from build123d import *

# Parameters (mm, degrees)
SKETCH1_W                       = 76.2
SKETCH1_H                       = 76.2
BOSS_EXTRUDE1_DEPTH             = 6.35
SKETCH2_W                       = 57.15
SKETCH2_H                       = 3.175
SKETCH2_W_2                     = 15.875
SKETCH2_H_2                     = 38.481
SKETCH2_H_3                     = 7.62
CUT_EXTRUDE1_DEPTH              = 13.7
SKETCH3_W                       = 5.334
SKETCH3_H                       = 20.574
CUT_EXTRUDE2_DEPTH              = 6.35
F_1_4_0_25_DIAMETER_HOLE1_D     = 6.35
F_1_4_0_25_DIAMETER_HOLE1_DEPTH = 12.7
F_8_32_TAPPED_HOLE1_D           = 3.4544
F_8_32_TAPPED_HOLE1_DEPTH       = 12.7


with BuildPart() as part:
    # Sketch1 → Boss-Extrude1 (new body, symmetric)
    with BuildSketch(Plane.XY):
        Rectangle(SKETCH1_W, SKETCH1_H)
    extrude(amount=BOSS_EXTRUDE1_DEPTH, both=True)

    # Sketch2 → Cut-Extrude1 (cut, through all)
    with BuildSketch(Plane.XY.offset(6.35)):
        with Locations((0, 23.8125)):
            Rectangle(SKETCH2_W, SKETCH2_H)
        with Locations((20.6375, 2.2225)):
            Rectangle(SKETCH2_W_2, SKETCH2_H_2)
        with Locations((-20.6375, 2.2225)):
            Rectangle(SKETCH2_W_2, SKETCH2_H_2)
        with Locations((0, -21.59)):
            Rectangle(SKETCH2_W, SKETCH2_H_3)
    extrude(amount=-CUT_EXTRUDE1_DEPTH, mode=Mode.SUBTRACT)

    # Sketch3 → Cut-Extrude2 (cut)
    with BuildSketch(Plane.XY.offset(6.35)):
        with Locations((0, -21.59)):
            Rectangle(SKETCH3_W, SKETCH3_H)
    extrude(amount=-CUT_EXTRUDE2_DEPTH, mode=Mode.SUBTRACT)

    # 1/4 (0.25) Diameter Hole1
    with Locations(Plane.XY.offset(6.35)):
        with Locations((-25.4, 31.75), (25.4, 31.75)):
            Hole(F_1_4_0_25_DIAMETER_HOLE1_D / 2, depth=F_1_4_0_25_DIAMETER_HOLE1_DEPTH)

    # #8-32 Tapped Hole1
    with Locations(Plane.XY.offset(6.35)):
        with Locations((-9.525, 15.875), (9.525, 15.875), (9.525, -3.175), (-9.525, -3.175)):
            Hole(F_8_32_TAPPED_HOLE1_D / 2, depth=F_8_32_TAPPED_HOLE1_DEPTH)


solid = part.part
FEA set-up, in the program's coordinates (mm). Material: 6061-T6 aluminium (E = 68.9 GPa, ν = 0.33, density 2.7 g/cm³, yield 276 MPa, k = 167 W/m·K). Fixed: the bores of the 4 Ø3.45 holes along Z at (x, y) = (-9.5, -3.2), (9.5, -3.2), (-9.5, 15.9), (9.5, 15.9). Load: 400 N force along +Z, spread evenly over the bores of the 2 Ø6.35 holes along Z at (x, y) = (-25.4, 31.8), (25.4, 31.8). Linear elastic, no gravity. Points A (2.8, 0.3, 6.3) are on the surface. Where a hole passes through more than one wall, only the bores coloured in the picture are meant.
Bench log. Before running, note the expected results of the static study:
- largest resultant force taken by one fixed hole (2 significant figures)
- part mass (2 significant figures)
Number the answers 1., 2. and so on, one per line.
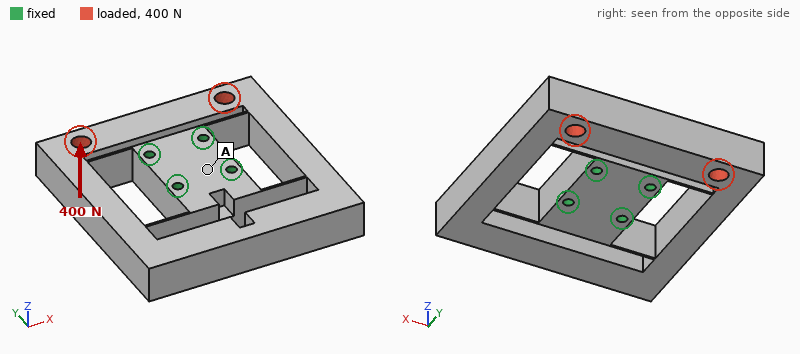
1. 270 N
2. 130 g
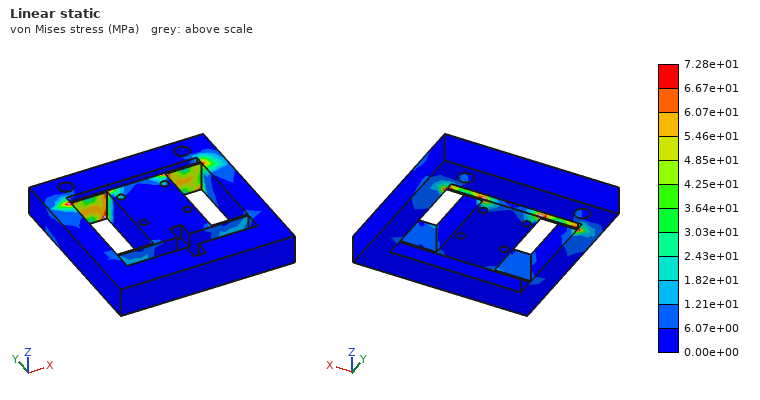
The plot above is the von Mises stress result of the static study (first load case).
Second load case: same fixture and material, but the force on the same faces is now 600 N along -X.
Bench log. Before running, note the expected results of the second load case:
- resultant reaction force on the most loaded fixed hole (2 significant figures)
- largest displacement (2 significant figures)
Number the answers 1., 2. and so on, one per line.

1. 400 N
2. 36 µm
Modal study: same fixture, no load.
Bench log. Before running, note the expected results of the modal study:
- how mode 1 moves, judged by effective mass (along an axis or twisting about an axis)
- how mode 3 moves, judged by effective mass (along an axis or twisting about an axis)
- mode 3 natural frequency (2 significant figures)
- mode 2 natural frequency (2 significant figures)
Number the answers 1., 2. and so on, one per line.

1. along Y
2. twisting about Z
3. 1700 Hz
4. 1600 Hz
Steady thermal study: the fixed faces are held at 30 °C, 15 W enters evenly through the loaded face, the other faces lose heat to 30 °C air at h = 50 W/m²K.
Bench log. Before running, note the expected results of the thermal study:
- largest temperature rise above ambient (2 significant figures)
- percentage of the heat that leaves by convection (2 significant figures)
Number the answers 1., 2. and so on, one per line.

1. 21 K
2. 67 %
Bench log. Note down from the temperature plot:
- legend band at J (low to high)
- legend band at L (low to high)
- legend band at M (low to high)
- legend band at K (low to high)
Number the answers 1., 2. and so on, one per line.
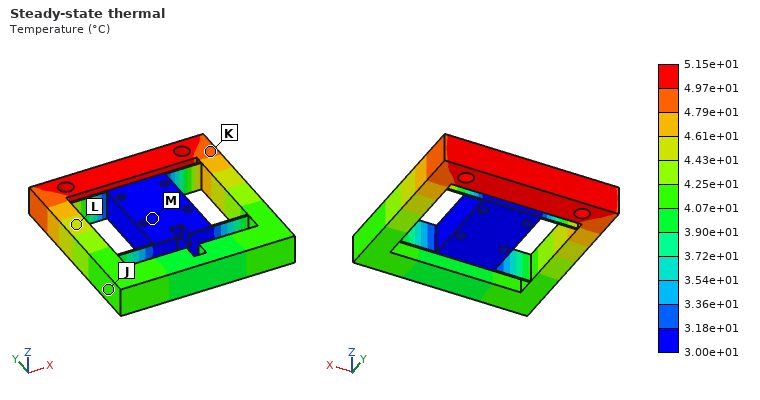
1. 4.07e+01 to 4.25e+01 °C
2. 4.43e+01 to 4.61e+01 °C
3. 3.00e+01 to 3.18e+01 °C
4. 4.79e+01 to 4.97e+01 °C
